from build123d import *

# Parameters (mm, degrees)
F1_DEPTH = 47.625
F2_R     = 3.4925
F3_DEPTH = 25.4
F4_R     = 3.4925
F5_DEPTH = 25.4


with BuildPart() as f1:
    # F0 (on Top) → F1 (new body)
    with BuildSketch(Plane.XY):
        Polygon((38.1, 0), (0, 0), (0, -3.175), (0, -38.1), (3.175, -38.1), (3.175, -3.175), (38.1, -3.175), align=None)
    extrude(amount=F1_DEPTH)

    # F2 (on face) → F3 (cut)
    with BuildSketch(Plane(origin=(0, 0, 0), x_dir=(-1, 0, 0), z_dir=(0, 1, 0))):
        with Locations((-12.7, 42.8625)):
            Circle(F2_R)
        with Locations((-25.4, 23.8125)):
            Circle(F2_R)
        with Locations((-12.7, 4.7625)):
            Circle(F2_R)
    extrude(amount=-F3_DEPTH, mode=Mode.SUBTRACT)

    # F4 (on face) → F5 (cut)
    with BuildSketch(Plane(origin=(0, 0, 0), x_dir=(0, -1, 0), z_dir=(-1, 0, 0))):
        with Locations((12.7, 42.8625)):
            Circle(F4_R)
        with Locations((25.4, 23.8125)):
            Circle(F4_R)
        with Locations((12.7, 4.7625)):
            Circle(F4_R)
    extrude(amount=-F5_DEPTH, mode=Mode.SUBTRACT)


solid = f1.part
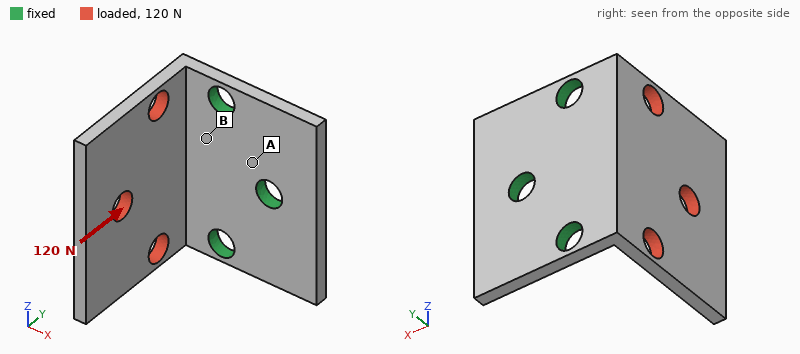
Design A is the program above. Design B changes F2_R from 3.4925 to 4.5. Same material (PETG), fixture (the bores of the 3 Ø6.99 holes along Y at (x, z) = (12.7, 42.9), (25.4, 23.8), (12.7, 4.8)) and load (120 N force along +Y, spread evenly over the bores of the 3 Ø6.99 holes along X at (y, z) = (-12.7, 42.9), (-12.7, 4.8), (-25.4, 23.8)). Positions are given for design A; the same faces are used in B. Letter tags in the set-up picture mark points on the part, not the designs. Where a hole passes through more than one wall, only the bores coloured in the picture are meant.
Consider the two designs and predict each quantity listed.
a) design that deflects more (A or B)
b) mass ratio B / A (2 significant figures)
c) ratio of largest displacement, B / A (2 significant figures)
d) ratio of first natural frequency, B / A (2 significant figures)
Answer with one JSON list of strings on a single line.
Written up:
["A", "0.98", "0.76", "1.0"]
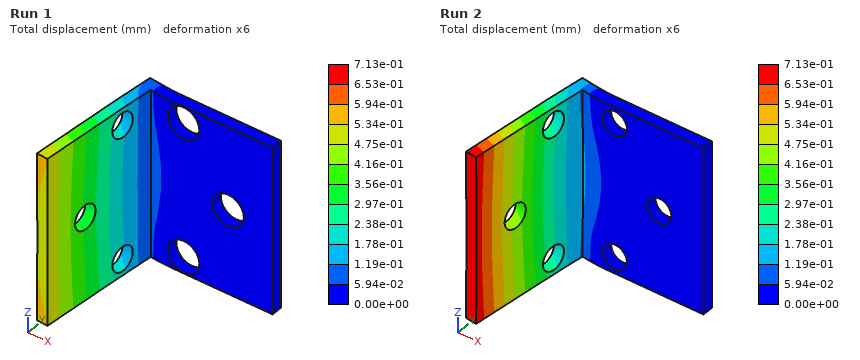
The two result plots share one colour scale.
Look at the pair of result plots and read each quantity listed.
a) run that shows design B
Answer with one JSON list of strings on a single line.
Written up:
["Run 1"]
